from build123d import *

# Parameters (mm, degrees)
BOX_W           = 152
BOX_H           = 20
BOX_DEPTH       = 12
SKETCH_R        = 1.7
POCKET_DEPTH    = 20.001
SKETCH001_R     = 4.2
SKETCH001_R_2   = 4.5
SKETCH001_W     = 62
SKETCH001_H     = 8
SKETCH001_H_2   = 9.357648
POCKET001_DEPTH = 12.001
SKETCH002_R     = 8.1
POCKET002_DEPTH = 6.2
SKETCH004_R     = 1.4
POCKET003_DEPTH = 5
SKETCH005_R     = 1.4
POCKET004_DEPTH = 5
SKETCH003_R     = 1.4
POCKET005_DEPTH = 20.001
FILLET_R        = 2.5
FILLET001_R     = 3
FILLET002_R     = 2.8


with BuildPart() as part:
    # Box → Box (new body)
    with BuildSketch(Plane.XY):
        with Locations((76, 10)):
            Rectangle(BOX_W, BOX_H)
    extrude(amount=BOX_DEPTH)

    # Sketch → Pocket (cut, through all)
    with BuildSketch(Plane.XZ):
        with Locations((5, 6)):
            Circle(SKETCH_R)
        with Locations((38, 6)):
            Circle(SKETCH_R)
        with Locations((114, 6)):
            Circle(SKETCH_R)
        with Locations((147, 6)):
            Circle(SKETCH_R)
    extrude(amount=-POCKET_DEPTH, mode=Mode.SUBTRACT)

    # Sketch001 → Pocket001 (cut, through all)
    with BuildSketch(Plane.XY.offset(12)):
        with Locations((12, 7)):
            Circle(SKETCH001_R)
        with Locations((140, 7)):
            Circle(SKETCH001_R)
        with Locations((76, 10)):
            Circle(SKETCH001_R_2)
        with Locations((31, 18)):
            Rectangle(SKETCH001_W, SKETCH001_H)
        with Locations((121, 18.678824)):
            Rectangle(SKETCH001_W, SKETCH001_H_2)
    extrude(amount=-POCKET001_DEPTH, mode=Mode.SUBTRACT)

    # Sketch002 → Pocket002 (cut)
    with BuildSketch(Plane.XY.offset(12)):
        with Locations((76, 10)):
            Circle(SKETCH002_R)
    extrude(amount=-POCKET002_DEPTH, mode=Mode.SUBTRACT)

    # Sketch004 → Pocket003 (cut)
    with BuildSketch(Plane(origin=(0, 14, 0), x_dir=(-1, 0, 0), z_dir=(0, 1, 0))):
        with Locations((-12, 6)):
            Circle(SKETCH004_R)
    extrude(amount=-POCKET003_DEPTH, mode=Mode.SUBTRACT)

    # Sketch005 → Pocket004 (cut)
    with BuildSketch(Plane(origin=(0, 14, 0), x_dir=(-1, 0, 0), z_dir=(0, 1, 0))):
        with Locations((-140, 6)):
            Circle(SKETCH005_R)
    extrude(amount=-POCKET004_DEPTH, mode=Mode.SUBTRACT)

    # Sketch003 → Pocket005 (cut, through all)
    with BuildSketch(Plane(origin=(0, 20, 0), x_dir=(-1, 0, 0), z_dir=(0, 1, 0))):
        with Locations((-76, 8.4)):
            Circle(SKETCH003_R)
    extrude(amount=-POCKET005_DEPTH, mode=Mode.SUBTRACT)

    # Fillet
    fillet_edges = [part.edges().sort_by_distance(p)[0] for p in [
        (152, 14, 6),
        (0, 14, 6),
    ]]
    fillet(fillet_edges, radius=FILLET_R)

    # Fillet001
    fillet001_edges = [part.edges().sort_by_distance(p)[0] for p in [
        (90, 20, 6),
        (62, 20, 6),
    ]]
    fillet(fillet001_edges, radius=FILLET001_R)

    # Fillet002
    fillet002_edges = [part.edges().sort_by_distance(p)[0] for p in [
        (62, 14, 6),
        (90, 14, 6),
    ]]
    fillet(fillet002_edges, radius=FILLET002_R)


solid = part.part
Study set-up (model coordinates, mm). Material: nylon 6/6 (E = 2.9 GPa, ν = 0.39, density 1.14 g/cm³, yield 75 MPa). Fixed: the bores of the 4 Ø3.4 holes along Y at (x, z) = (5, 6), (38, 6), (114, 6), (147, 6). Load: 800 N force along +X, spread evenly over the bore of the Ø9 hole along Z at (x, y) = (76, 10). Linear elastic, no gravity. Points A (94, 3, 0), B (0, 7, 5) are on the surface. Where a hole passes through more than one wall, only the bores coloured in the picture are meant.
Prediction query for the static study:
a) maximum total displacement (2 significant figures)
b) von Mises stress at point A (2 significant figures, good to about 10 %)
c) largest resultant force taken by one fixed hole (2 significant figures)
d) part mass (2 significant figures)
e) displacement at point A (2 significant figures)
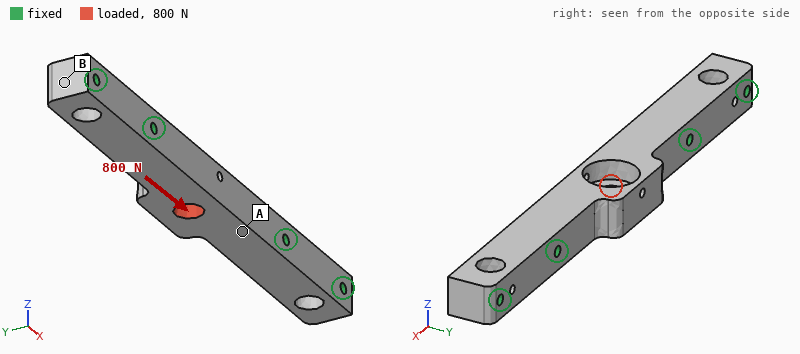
49 µm
3.0 MPa
390 N
27 g
20 µm
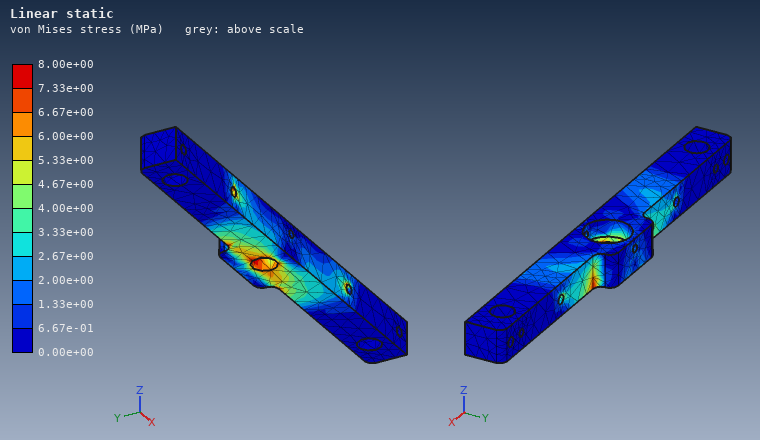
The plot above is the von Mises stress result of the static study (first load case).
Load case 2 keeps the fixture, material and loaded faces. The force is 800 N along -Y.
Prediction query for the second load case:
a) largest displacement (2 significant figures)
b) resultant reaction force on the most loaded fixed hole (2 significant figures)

0.33 mm
430 N
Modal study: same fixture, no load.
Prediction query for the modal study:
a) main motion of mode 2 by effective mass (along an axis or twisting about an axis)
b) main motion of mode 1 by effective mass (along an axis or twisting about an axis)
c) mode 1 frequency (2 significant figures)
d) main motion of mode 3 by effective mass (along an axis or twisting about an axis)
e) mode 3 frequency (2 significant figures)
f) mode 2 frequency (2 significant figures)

along Y
along Z
2200 Hz
twisting about X
4600 Hz
3500 Hz
